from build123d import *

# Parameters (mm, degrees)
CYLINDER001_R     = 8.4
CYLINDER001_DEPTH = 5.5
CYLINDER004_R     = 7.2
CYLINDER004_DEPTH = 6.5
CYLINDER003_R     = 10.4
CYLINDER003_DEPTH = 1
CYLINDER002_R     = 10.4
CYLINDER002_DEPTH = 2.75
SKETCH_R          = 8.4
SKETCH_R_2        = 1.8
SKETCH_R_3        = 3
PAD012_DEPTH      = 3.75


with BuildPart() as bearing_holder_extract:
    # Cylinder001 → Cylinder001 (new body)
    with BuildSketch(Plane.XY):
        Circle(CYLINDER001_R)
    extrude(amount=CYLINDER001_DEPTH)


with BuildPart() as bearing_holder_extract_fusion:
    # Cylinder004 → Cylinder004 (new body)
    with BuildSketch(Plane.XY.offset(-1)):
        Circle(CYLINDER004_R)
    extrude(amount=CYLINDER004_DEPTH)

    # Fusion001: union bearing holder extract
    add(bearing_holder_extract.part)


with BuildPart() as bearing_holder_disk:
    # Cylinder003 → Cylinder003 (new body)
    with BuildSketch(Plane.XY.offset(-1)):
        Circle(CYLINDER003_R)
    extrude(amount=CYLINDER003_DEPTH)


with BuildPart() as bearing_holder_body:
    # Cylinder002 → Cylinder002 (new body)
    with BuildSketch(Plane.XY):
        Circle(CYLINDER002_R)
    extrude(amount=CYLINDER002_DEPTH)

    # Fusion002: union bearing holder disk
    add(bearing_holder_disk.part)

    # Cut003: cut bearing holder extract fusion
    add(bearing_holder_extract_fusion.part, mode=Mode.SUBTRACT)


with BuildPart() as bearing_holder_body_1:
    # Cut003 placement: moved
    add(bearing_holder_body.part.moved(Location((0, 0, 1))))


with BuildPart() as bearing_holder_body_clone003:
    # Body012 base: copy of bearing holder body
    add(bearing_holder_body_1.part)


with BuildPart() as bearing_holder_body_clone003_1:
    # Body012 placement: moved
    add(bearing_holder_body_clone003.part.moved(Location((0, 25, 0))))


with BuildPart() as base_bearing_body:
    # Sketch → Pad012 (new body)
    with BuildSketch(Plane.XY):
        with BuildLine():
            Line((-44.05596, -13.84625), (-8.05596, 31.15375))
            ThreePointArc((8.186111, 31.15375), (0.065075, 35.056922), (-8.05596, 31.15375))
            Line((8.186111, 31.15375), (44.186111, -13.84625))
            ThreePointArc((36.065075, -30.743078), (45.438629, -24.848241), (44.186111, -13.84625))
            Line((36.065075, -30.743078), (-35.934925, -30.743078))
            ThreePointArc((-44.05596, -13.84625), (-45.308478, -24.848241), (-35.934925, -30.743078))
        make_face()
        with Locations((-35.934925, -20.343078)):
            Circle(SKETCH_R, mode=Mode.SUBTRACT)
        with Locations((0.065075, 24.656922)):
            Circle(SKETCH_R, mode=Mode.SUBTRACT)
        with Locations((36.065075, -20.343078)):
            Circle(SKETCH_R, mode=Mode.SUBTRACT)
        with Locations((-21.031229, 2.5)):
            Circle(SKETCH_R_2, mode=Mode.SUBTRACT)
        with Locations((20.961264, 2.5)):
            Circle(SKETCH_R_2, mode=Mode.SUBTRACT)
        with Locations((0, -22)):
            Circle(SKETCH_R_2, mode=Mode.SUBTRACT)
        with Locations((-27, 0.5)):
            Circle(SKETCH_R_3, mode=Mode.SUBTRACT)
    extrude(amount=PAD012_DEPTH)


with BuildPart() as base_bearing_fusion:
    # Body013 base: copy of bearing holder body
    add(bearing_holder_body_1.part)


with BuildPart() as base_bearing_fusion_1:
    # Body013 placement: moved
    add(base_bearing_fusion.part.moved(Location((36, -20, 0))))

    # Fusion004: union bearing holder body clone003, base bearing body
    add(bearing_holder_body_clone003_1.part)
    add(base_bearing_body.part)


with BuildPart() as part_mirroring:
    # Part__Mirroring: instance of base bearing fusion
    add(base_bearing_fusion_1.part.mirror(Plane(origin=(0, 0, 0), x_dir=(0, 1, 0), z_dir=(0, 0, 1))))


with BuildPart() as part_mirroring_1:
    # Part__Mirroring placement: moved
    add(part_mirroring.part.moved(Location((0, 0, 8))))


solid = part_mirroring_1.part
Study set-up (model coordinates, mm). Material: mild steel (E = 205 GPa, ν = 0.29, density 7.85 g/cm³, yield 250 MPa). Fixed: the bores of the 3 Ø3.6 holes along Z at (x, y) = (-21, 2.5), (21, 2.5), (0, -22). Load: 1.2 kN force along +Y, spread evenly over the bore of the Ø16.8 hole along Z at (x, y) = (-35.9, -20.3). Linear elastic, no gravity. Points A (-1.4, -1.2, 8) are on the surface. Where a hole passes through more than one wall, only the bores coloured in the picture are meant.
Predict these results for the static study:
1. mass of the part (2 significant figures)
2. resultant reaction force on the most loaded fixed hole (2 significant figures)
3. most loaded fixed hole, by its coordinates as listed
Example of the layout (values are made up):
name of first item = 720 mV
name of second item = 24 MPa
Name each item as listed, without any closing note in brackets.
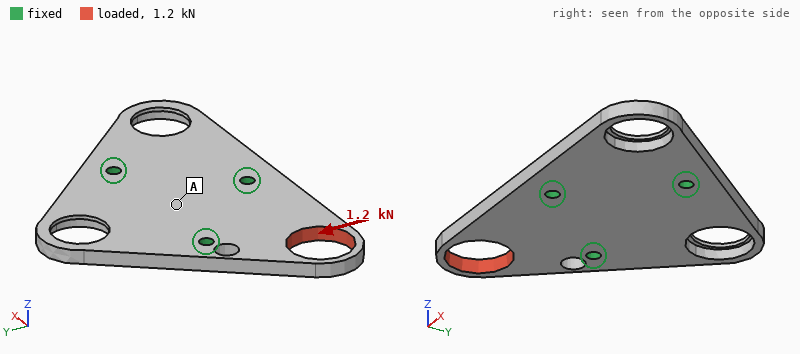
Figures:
mass of the part = 95 g
resultant reaction force on the most loaded fixed hole = 1.3 kN
most loaded fixed hole, by its coordinates as listed = (-21, 2.5)
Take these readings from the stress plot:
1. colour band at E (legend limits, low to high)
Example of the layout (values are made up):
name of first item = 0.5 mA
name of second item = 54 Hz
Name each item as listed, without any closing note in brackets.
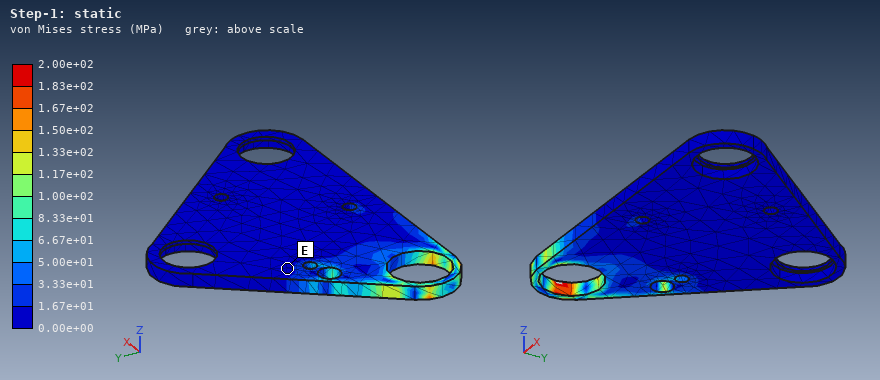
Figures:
colour band at E = 0.00e+00 to 1.67e+01 MPa
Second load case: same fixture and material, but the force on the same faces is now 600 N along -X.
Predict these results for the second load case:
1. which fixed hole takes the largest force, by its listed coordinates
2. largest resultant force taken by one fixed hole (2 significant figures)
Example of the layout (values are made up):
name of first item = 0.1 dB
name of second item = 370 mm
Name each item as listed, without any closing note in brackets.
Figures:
which fixed hole takes the largest force, by its listed coordinates = (0, -22)
largest resultant force taken by one fixed hole = 430 N
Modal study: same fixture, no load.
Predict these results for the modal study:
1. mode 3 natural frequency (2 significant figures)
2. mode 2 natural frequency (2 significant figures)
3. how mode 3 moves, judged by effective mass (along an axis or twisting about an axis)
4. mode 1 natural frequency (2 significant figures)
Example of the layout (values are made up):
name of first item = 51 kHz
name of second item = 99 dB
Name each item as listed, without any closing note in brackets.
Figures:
mode 3 natural frequency = 4600 Hz
mode 2 natural frequency = 3900 Hz
how mode 3 moves, judged by effective mass = along Z
mode 1 natural frequency = 3900 Hz
